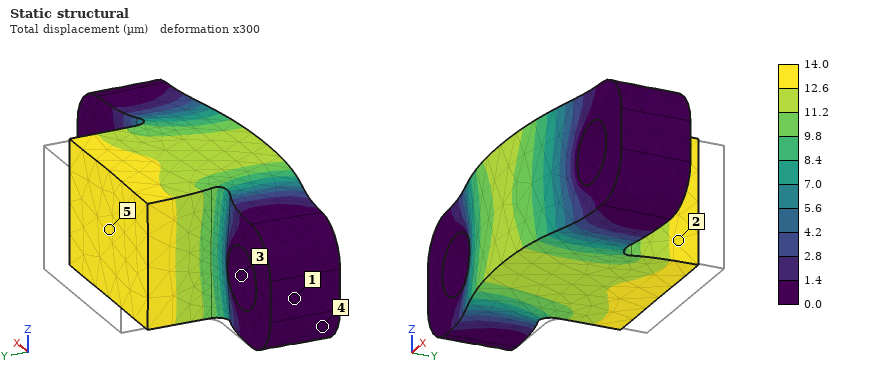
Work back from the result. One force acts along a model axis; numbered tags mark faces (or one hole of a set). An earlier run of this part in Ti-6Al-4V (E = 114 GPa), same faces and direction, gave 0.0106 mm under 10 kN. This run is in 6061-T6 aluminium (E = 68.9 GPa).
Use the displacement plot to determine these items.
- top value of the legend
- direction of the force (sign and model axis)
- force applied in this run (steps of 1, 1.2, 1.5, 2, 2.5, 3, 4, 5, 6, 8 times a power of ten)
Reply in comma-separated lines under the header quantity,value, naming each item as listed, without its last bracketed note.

quantity,value
top value of the legend,14.0 µm
direction of the force,-Y
force applied in this run,8 kN
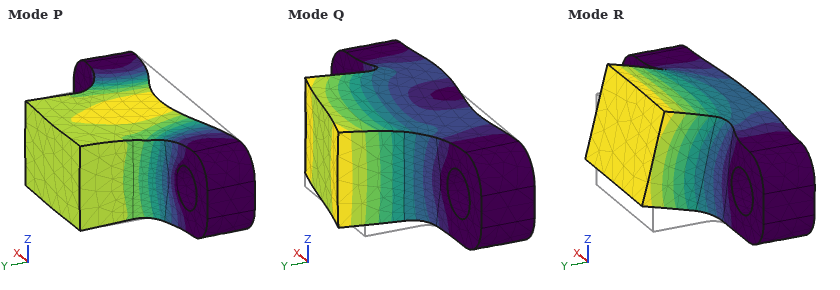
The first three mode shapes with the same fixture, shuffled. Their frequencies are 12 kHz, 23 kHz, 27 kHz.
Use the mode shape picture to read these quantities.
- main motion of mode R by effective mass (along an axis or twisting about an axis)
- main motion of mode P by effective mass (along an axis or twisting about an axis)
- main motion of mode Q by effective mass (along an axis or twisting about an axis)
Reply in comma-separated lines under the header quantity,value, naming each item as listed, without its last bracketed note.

quantity,value
main motion of mode R by effective mass,along Z
main motion of mode P by effective mass,along Y
main motion of mode Q by effective mass,along X
